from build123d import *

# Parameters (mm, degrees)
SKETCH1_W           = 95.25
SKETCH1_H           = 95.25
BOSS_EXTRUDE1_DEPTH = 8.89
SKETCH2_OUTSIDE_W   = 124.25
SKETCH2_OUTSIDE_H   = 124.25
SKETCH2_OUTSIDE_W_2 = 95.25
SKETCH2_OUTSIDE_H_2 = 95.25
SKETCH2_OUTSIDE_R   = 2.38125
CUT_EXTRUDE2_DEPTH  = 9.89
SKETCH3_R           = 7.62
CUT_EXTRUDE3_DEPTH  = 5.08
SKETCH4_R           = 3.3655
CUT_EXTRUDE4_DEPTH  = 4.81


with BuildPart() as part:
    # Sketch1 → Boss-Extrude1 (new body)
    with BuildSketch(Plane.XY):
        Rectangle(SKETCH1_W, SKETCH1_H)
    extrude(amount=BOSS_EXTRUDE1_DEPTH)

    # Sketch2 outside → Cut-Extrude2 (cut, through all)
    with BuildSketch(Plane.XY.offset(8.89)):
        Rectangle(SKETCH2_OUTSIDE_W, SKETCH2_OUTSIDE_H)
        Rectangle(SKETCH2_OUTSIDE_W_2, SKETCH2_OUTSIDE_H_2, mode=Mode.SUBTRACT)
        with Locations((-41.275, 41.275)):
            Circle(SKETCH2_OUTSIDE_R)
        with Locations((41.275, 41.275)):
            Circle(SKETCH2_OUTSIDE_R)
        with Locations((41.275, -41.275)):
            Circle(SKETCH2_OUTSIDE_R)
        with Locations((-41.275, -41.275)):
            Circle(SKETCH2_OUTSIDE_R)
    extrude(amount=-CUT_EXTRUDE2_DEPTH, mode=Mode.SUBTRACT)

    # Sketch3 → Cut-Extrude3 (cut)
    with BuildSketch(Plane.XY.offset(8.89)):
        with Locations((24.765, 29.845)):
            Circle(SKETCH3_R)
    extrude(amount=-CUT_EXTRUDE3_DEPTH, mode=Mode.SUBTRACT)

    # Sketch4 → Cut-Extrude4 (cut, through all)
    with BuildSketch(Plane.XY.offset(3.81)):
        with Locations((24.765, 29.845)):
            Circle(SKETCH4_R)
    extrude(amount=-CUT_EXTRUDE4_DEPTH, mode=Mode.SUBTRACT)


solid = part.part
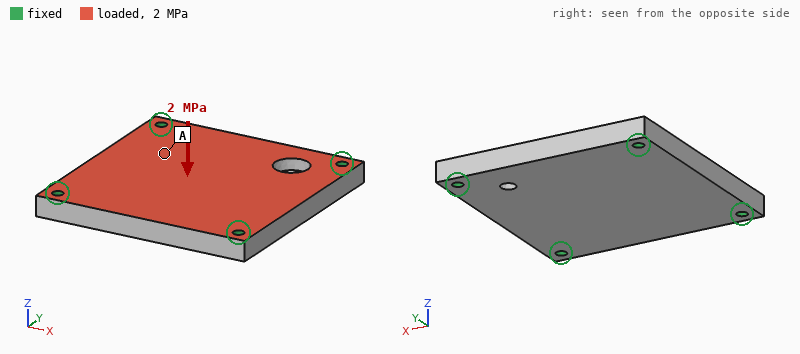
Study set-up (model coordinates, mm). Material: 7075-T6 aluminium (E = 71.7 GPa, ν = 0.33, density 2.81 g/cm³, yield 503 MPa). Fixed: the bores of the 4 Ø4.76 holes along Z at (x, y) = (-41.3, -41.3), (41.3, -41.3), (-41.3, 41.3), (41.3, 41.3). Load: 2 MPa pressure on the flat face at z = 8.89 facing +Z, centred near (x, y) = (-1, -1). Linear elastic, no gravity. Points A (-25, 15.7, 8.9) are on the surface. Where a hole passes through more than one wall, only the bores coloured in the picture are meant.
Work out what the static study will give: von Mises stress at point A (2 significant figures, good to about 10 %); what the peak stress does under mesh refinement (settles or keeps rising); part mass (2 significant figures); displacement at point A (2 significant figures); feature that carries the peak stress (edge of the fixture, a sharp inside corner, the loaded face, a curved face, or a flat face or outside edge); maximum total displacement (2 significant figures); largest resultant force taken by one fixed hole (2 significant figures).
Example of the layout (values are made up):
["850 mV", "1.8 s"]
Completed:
["41 MPa", "keeps rising", "220 g", "0.13 mm", "edge of the fixture", "0.19 mm", "4.5 kN"]
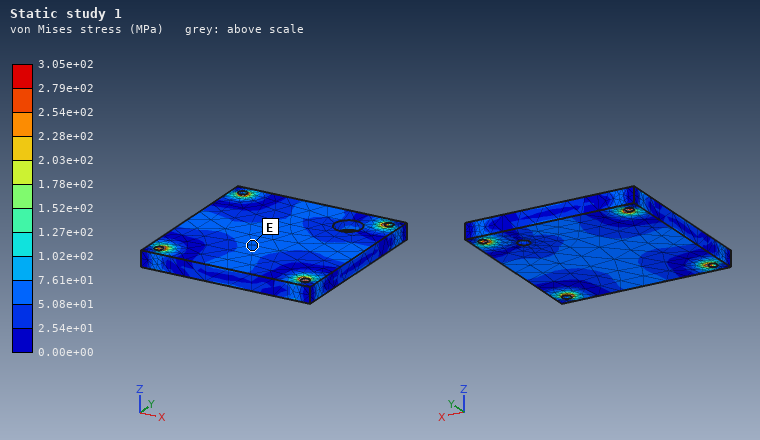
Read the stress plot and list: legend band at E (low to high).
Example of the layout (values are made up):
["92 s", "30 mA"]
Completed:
["5.08e+01 to 7.61e+01 MPa"]
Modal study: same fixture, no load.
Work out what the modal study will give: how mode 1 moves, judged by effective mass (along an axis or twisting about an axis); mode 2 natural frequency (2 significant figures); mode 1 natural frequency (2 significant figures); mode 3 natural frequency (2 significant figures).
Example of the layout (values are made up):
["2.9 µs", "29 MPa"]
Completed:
["along Z", "6700 Hz", "3900 Hz", "6700 Hz"]
